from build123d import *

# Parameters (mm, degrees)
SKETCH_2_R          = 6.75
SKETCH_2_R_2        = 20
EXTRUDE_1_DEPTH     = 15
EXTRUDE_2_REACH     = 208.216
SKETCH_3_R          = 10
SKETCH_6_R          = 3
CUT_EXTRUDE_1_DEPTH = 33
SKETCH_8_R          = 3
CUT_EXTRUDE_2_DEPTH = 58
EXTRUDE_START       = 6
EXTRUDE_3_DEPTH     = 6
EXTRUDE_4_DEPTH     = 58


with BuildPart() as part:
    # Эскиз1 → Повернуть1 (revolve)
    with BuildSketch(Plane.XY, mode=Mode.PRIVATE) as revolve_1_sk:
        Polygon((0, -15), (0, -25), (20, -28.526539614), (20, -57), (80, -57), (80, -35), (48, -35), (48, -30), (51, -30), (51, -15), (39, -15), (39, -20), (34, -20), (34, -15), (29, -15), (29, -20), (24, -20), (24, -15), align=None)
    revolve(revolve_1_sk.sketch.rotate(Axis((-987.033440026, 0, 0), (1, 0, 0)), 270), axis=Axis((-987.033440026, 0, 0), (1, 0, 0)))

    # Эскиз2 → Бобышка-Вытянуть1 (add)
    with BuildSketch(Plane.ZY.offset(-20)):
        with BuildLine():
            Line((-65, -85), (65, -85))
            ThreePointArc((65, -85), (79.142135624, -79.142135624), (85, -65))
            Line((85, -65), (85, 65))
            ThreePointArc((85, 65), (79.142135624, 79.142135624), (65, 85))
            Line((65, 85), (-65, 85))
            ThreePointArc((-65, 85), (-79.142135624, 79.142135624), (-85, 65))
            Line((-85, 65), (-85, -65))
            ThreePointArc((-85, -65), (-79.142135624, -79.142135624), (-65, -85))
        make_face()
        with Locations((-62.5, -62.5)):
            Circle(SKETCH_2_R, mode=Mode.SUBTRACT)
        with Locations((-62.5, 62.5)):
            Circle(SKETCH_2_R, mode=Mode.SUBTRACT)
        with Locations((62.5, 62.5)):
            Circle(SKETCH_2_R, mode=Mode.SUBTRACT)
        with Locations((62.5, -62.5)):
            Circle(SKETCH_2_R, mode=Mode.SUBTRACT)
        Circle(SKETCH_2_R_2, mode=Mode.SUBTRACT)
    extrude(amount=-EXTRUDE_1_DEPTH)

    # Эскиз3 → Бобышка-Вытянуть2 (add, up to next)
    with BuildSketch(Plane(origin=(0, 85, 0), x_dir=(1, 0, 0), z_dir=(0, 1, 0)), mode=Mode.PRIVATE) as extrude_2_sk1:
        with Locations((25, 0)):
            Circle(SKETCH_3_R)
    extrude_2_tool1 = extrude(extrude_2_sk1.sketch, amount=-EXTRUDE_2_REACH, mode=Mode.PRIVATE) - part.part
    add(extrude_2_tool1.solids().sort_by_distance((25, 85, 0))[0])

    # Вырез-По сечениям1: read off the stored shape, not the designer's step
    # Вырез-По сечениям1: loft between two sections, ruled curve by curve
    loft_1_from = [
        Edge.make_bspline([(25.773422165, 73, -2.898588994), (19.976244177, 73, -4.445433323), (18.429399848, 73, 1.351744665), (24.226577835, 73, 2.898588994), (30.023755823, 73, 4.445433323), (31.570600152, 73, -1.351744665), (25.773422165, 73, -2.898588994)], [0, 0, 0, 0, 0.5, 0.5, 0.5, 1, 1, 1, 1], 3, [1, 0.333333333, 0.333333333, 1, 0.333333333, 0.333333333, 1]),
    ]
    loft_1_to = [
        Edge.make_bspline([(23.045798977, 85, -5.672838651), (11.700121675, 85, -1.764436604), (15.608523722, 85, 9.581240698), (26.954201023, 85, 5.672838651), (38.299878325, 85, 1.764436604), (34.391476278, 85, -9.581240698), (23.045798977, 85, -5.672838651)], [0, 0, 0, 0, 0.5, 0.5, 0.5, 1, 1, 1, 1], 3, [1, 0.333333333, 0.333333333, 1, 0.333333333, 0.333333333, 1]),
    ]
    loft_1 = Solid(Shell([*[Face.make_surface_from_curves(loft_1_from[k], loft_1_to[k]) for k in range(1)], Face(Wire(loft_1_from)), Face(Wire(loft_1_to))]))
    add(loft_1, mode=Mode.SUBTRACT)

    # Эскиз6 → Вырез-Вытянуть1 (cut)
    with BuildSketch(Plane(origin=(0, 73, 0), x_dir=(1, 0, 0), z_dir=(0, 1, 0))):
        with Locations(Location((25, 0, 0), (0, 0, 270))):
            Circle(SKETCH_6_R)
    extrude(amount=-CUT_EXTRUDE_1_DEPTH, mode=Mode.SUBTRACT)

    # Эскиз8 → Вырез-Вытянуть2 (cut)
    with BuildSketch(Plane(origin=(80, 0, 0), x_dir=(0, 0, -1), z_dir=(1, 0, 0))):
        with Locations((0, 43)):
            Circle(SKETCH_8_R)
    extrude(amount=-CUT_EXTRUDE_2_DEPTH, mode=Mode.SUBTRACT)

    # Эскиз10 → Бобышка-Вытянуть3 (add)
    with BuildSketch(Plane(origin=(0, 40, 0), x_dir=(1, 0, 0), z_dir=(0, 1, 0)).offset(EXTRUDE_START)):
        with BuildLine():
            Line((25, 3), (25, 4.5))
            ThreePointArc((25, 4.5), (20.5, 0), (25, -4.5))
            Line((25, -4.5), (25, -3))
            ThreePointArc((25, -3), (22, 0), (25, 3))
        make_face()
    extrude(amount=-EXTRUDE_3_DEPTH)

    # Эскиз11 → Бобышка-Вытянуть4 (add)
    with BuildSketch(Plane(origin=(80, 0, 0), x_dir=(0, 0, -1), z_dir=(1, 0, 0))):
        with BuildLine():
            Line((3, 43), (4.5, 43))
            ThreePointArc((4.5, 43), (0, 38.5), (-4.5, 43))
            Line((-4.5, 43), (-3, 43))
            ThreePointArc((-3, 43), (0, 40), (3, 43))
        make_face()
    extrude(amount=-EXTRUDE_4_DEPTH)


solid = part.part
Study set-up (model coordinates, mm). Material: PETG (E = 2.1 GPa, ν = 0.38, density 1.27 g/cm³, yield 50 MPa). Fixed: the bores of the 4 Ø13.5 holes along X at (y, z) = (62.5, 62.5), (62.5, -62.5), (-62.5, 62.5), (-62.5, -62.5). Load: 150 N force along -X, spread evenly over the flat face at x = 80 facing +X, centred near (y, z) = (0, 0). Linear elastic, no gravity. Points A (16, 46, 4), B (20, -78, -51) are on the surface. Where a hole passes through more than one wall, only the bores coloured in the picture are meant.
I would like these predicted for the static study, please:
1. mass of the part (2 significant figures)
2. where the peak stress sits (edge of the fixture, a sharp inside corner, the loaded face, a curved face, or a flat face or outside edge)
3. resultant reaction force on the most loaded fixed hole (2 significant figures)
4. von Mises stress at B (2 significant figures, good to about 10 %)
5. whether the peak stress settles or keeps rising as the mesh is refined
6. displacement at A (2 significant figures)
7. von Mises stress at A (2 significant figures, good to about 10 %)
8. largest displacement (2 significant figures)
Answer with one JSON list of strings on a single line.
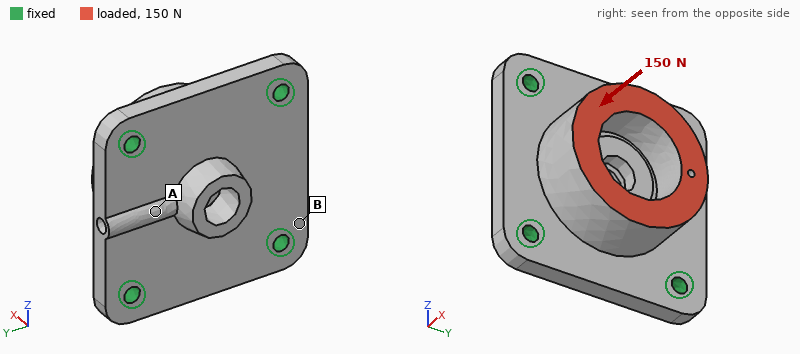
["980 g", "edge of the fixture", "40 N", "0.083 MPa", "keeps rising", "7.3 µm", "0.038 MPa", "7.9 µm"]
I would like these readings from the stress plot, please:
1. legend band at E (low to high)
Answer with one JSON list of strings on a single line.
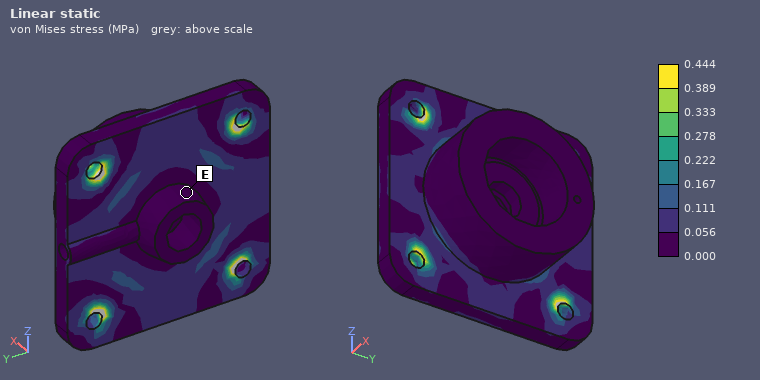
["0.000 to 0.056 MPa"]
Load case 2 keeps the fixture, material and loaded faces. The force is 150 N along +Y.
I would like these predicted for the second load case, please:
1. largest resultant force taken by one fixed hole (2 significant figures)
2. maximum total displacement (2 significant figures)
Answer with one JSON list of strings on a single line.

["54 N", "14 µm"]
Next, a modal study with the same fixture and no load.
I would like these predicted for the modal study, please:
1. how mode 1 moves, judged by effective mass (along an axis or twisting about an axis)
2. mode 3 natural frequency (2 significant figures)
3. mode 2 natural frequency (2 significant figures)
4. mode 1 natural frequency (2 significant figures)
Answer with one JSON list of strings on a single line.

["along X", "1000 Hz", "1000 Hz", "820 Hz"]
